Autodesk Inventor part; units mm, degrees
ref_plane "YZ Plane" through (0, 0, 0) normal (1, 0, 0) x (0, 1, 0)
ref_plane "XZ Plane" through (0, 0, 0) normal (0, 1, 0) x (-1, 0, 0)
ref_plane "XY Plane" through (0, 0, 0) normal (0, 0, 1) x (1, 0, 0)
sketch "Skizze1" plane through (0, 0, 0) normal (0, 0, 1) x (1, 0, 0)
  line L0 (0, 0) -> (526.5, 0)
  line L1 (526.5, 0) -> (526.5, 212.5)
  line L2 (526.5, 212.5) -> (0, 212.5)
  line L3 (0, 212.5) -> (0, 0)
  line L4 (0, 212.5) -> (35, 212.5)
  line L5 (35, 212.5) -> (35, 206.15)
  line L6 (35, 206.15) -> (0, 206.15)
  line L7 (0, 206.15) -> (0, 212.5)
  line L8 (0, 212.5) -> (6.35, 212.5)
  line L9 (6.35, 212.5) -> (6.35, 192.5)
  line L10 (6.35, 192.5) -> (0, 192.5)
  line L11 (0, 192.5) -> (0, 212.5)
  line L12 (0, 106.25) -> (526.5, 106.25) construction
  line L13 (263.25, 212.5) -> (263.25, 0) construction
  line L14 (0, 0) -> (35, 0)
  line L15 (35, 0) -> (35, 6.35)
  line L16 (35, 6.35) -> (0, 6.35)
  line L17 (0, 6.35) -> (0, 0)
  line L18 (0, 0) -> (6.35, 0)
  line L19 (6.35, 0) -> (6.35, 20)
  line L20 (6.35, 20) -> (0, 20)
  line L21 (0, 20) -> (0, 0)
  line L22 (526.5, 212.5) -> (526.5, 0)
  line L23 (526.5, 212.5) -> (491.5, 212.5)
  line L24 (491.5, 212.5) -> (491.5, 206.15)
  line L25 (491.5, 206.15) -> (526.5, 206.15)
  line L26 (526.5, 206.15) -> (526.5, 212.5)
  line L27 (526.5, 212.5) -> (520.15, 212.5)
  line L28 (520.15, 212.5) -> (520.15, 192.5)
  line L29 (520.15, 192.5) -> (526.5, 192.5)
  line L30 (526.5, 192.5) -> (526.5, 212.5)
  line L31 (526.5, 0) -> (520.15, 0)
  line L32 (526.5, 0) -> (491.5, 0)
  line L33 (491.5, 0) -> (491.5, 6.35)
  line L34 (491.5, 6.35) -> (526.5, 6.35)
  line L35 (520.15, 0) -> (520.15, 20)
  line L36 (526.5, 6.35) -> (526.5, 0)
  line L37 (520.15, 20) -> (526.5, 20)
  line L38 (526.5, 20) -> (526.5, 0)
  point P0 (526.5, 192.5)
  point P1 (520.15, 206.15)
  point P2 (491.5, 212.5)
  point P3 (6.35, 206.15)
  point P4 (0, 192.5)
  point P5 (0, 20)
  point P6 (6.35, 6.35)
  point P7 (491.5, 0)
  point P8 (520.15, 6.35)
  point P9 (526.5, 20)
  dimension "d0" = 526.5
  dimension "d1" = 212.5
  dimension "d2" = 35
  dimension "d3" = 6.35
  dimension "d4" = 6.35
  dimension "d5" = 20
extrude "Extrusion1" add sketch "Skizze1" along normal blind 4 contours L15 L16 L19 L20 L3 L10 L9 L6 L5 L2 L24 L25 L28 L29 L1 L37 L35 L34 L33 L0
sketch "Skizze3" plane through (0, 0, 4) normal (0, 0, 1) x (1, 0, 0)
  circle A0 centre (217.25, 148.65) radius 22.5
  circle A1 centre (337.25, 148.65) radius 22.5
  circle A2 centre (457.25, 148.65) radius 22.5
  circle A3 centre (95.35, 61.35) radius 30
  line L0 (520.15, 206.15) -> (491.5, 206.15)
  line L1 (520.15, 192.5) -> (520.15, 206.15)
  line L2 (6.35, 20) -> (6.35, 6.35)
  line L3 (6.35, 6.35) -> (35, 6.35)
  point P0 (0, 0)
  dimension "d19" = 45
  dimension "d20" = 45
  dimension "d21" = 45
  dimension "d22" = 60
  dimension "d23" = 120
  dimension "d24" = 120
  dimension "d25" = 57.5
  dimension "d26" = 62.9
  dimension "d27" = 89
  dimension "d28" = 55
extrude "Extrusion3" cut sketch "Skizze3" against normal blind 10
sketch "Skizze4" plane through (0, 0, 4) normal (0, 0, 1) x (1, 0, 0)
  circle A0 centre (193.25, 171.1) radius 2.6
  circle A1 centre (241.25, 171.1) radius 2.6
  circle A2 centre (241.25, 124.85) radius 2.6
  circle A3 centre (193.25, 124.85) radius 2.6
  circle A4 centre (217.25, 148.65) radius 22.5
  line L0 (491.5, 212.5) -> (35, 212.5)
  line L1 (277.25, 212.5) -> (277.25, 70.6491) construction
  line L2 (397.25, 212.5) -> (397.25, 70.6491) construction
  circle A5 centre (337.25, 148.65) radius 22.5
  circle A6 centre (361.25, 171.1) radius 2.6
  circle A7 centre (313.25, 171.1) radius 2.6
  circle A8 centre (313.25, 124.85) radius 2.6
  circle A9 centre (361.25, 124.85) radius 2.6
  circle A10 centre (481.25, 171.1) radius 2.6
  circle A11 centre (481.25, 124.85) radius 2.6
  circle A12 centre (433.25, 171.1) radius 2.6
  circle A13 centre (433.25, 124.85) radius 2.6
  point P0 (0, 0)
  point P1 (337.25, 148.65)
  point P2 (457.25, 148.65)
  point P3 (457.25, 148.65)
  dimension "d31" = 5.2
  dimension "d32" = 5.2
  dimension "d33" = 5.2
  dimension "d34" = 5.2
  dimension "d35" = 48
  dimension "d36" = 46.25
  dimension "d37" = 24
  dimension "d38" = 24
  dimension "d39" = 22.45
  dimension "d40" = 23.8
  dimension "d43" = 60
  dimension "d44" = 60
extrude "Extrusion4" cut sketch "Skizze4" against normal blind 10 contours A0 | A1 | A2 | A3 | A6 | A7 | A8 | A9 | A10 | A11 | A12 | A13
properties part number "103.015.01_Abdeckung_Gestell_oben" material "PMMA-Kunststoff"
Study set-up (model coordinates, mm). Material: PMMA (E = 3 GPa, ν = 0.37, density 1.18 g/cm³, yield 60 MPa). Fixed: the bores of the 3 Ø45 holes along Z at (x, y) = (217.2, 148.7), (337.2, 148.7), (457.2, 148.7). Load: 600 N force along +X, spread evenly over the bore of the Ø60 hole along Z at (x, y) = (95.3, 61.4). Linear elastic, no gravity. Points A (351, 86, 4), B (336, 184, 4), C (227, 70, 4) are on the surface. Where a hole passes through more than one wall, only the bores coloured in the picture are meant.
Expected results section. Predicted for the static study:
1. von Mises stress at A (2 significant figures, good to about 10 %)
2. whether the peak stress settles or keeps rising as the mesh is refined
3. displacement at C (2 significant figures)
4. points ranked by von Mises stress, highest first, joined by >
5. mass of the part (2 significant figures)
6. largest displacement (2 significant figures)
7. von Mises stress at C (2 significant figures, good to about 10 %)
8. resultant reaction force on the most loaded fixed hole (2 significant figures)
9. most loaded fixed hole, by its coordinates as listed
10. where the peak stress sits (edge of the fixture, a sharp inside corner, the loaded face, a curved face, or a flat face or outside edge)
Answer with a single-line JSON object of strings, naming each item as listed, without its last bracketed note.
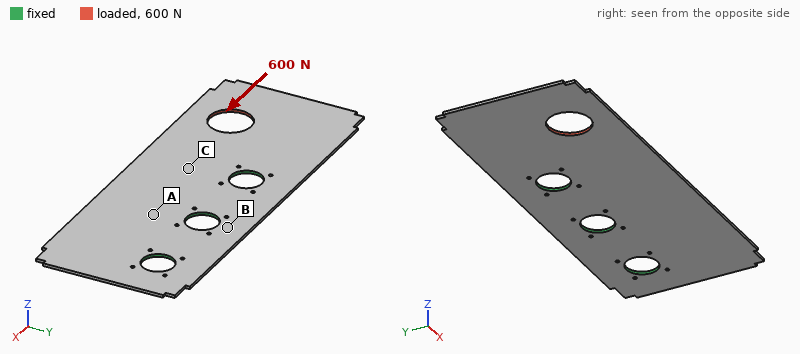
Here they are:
{"von Mises stress at A": "0.57 MPa", "whether the peak stress settles or keeps rising as the mesh is refined": "keeps rising", "displacement at C": "0.042 mm", "points ranked by von Mises stress, highest first, joined by >": "C > A > B", "mass of the part": "490 g", "largest displacement": "0.21 mm", "von Mises stress at C": "1.0 MPa", "resultant reaction force on the most loaded fixed hole": "390 N", "most loaded fixed hole, by its coordinates as listed": "(217.2, 148.7)", "where the peak stress sits": "a sharp inside corner"}
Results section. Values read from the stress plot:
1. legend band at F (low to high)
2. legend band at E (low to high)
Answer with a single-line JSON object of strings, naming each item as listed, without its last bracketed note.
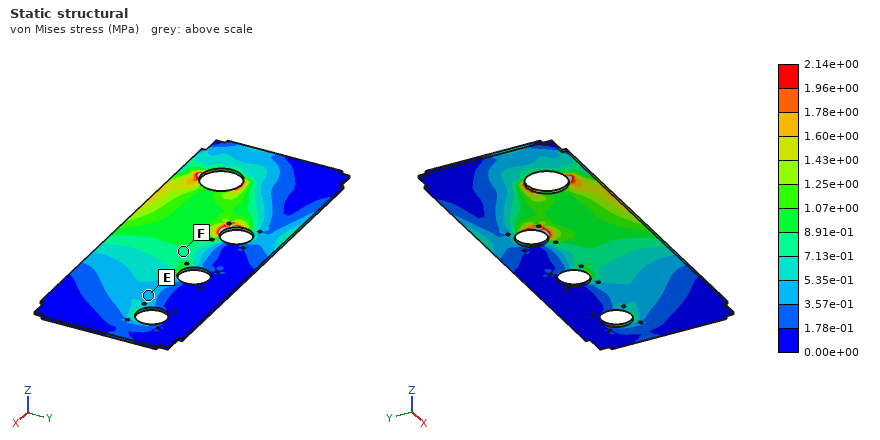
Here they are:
{"legend band at F": "7.13e-01 to 8.91e-01 MPa", "legend band at E": "3.57e-01 to 5.35e-01 MPa"}
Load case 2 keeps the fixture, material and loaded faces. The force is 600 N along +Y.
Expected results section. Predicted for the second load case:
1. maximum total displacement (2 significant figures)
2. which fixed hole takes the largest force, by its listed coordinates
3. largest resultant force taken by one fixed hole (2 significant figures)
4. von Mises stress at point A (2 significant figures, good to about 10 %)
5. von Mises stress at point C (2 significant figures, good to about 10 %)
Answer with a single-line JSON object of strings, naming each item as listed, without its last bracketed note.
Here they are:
{"maximum total displacement": "0.36 mm", "which fixed hole takes the largest force, by its listed coordinates": "(217.2, 148.7)", "largest resultant force taken by one fixed hole": "870 N", "von Mises stress at point A": "0.65 MPa", "von Mises stress at point C": "1.0 MPa"}
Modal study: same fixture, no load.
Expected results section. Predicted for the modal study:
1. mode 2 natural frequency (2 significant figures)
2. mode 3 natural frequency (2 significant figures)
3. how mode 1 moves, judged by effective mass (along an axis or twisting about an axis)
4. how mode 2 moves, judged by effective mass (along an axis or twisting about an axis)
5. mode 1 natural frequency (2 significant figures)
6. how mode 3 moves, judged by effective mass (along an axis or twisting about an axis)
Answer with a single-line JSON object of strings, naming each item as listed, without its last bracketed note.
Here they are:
{"mode 2 natural frequency": "46 Hz", "mode 3 natural frequency": "66 Hz", "how mode 1 moves, judged by effective mass": "along Z", "how mode 2 moves, judged by effective mass": "twisting about X", "mode 1 natural frequency": "24 Hz", "how mode 3 moves, judged by effective mass": "along Z"}
